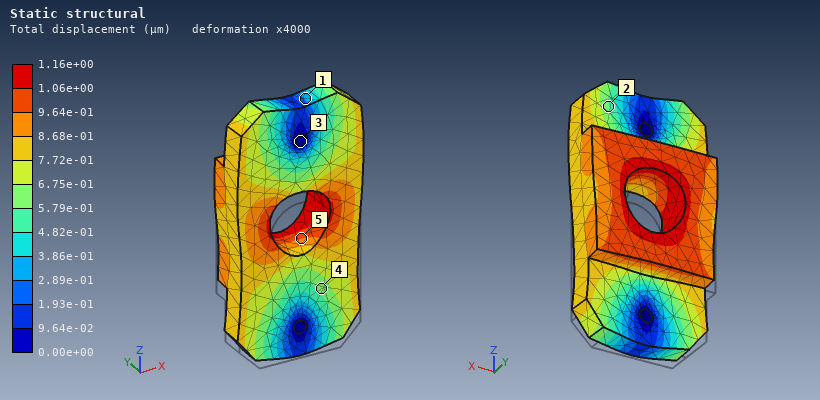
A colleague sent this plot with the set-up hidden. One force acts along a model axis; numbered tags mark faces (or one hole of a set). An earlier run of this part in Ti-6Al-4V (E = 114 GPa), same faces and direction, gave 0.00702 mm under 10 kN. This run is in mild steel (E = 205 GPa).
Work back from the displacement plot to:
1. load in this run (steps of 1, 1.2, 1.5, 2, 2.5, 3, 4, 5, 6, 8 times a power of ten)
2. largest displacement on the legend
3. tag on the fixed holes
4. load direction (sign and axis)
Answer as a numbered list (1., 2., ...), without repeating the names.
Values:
1. 3 kN
2. 1.16e+00 µm
3. 3
4. +Z
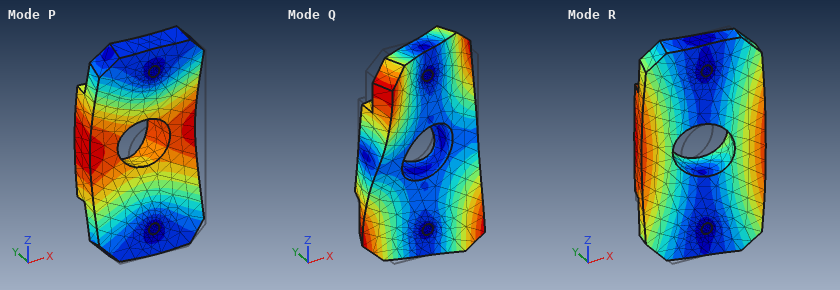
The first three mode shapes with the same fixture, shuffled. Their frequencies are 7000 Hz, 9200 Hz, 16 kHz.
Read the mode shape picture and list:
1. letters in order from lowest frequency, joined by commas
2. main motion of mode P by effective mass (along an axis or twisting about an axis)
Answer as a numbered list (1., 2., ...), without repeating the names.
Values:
1. R, P, Q
2. along Y
